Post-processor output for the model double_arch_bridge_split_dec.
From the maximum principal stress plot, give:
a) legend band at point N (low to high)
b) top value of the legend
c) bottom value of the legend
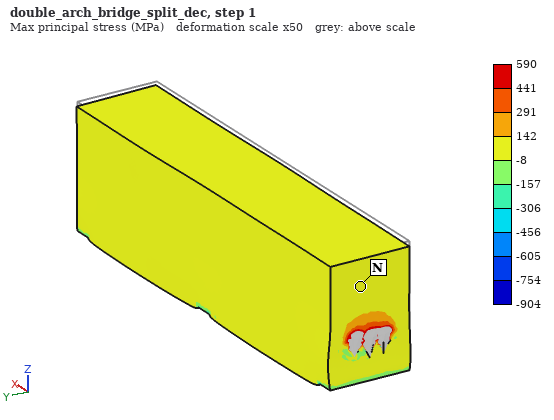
-8 to 142 MPa
590 MPa
-904 MPa
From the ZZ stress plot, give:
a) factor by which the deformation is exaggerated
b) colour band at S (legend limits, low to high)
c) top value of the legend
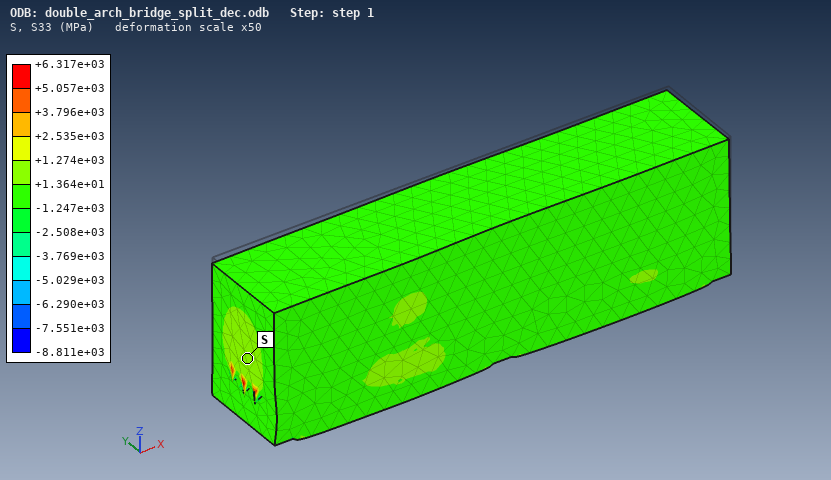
50
+1.364e+01 to +1.274e+03 MPa
+6.317e+03 MPa
